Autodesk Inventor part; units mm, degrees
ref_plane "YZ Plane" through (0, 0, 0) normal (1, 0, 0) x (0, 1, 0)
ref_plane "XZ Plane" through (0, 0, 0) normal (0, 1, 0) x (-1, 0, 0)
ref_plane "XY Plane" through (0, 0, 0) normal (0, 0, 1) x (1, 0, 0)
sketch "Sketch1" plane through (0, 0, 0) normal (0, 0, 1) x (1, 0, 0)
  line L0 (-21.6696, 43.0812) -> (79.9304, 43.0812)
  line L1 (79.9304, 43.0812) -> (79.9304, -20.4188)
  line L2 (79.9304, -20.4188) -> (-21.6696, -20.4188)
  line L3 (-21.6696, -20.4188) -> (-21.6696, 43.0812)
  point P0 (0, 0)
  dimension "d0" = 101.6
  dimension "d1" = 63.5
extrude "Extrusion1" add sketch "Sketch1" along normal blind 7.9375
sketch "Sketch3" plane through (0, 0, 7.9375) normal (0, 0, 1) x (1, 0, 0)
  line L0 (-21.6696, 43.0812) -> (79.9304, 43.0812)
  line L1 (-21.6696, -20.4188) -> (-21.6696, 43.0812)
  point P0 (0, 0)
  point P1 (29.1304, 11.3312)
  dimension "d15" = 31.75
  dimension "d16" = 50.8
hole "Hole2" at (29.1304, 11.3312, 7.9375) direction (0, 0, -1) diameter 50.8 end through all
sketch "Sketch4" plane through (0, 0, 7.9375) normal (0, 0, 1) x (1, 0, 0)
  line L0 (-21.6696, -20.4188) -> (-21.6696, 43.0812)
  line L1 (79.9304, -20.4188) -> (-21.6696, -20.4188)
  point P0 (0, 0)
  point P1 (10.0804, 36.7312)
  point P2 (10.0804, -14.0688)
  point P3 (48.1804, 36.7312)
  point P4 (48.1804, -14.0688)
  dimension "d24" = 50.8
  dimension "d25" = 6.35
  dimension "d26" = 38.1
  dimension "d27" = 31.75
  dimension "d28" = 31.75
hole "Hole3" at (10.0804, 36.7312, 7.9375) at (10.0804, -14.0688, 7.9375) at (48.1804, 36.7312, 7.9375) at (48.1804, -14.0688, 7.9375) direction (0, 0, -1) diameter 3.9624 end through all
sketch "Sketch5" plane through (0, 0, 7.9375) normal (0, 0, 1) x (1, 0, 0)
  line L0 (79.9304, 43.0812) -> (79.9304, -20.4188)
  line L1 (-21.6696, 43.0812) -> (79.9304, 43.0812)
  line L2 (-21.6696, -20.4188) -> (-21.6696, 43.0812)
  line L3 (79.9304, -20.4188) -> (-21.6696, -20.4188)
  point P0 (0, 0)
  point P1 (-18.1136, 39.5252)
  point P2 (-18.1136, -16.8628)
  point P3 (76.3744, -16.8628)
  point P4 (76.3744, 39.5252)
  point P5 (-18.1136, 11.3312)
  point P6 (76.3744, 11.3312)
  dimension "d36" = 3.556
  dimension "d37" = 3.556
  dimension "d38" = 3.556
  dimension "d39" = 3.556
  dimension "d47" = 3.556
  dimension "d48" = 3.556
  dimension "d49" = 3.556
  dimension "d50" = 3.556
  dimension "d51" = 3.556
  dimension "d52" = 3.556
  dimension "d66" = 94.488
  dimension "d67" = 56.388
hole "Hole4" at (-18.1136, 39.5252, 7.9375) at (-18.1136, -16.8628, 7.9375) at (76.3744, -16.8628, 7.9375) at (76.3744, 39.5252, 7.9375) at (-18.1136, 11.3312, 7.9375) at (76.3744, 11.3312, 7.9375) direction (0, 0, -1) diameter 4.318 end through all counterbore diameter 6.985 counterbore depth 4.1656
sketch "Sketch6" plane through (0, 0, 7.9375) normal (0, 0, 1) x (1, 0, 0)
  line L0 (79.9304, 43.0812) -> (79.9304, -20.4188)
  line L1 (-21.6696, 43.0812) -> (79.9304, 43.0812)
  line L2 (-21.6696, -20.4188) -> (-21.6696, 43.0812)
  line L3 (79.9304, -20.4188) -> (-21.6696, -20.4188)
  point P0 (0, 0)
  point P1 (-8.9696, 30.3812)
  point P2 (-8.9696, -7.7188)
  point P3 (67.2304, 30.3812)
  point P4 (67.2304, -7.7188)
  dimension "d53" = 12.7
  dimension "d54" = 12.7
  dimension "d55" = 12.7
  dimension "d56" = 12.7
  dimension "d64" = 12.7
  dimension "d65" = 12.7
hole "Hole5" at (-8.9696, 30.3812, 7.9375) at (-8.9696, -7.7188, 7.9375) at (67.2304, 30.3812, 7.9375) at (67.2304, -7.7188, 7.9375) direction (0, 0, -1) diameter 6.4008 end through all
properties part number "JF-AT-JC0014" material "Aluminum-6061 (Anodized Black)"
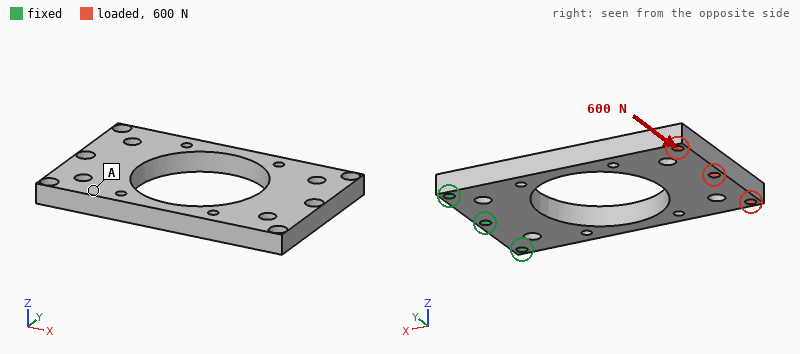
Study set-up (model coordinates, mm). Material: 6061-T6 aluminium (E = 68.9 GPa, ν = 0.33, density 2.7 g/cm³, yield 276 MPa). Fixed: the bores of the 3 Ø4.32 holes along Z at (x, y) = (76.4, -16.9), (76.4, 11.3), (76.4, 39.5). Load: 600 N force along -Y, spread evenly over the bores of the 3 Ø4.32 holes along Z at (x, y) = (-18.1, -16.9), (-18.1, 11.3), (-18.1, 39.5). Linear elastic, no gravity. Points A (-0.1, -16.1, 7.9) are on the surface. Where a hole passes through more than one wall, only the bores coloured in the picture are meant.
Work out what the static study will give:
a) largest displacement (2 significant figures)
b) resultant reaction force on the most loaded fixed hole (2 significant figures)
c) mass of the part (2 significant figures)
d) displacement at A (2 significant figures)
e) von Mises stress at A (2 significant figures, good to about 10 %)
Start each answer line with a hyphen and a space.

- 0.11 mm
- 1.0 kN
- 88 g
- 0.088 mm
- 5.8 MPa
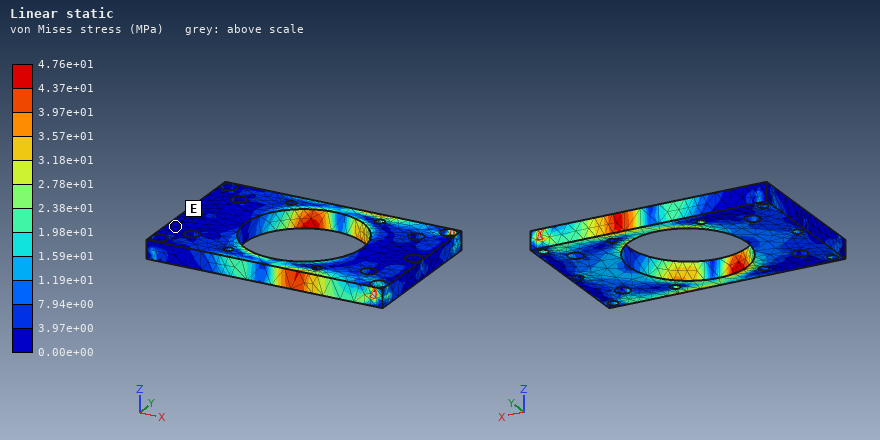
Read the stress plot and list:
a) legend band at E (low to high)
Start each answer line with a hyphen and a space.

- 0.00e+00 to 3.97e+00 MPa
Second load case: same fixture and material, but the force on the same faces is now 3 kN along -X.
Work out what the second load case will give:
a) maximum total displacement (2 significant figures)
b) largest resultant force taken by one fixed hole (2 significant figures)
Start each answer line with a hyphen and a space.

- 0.44 mm
- 1.3 kN
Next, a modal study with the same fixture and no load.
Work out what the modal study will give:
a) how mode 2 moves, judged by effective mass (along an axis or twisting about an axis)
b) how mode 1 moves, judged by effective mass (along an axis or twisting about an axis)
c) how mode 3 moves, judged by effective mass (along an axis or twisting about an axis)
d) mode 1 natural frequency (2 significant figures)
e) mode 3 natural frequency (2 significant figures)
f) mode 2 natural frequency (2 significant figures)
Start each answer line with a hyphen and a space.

- twisting about X
- along Z
- along Y
- 440 Hz
- 2100 Hz
- 1500 Hz
